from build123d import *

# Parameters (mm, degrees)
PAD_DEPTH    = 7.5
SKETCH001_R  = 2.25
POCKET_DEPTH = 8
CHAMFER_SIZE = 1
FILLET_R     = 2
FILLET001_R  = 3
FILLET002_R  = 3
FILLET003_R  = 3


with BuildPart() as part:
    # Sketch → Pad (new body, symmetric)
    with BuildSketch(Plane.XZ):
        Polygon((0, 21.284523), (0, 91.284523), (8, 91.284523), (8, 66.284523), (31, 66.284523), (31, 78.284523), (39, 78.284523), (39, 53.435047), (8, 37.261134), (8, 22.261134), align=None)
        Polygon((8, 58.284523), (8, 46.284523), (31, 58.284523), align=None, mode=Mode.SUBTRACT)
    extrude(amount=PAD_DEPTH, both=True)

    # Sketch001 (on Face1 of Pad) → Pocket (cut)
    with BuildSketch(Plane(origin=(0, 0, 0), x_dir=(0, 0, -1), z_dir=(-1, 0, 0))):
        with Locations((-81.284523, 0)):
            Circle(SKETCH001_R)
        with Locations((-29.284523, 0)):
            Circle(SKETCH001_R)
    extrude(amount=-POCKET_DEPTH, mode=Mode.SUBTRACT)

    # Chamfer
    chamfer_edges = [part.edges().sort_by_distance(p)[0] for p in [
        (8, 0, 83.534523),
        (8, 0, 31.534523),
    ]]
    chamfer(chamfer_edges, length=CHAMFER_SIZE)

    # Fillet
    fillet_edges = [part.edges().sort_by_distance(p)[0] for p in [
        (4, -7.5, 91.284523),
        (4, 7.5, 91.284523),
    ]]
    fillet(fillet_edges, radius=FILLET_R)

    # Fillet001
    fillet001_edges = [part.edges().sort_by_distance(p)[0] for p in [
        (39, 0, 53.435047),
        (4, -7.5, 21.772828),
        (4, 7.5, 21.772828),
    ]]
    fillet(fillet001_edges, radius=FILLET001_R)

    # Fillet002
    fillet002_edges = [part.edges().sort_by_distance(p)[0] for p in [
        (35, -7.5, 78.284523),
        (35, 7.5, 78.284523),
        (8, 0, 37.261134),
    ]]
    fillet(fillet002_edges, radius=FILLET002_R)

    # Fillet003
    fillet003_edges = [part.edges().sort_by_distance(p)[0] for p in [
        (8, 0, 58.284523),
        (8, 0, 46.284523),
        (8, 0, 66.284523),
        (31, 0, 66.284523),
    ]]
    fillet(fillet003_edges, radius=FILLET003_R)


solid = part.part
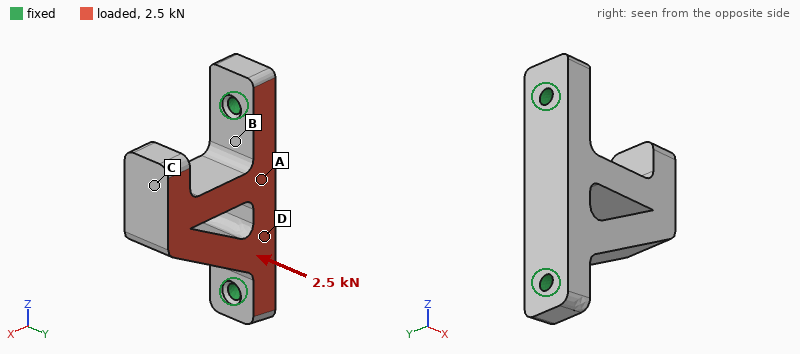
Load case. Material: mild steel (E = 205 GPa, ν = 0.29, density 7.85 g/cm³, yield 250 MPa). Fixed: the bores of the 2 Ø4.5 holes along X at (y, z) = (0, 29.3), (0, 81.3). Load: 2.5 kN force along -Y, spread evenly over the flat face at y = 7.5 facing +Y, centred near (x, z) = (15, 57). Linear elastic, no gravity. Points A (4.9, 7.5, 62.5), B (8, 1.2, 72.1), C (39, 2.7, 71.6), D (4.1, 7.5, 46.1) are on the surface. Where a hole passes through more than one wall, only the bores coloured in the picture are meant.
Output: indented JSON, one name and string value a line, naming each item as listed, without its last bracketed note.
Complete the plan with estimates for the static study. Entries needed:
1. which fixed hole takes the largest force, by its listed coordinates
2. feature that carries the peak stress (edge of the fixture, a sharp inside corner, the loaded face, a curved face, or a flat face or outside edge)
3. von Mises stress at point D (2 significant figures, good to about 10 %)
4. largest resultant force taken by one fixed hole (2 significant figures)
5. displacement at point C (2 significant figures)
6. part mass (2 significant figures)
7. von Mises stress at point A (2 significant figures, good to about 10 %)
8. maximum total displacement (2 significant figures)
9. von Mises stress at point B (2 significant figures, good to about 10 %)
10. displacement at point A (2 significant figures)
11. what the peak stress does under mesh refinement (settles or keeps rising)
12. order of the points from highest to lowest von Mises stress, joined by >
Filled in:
{
  "which fixed hole takes the largest force, by its listed coordinates": "(0, 81.3)",
  "feature that carries the peak stress": "edge of the fixture",
  "von Mises stress at point D": "27 MPa",
  "largest resultant force taken by one fixed hole": "1.3 kN",
  "displacement at point C": "61 µm",
  "part mass": "140 g",
  "von Mises stress at point A": "39 MPa",
  "maximum total displacement": "63 µm",
  "von Mises stress at point B": "92 MPa",
  "displacement at point A": "12 µm",
  "what the peak stress does under mesh refinement": "keeps rising",
  "order of the points from highest to lowest von Mises stress, joined by >": "B > A > D > C"
}
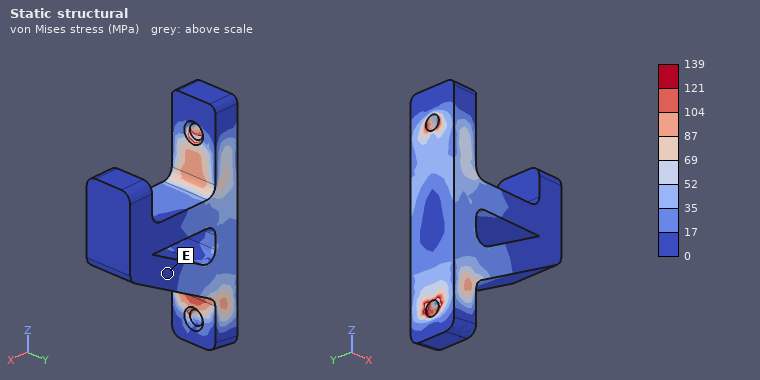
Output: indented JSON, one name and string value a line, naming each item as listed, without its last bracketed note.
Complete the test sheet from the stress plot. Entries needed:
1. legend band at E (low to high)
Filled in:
{
  "legend band at E": "0 to 17 MPa"
}
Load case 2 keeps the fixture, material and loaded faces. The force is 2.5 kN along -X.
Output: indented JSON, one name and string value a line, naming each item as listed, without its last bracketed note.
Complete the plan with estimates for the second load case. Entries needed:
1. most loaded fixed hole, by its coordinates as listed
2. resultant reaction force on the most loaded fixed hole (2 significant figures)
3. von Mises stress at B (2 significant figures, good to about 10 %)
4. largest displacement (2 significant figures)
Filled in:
{
  "most loaded fixed hole, by its coordinates as listed": "(0, 81.3)",
  "resultant reaction force on the most loaded fixed hole": "1.4 kN",
  "von Mises stress at B": "39 MPa",
  "largest displacement": "34 µm"
}
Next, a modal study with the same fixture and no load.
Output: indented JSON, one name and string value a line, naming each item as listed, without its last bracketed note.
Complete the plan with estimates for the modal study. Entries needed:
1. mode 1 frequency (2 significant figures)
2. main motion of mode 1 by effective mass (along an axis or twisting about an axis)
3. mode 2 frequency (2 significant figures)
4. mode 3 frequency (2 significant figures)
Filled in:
{
  "mode 1 frequency": "3300 Hz",
  "main motion of mode 1 by effective mass": "along Y",
  "mode 2 frequency": "7000 Hz",
  "mode 3 frequency": "11 kHz"
}
